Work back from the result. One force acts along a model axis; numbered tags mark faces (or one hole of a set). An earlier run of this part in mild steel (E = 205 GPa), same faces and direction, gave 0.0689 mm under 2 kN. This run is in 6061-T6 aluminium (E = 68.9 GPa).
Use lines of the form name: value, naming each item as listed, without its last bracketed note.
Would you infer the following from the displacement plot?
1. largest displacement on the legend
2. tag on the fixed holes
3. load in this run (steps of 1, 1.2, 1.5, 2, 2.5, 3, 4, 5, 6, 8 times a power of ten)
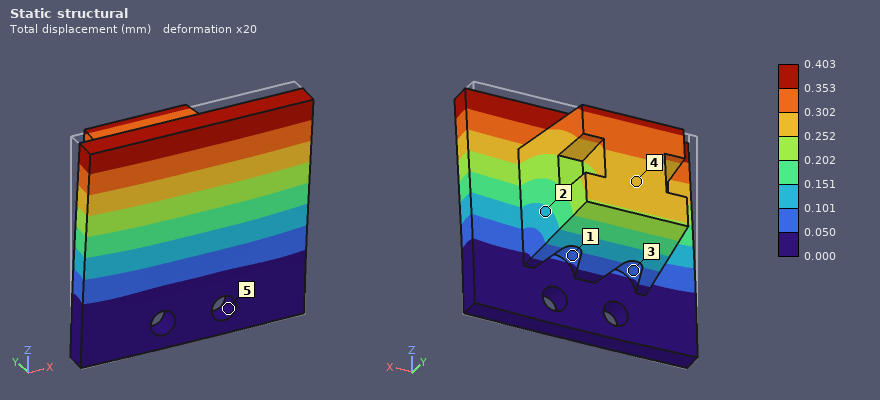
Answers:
largest displacement on the legend: 0.403 mm
tag on the fixed holes: 5
load in this run: 4 kN
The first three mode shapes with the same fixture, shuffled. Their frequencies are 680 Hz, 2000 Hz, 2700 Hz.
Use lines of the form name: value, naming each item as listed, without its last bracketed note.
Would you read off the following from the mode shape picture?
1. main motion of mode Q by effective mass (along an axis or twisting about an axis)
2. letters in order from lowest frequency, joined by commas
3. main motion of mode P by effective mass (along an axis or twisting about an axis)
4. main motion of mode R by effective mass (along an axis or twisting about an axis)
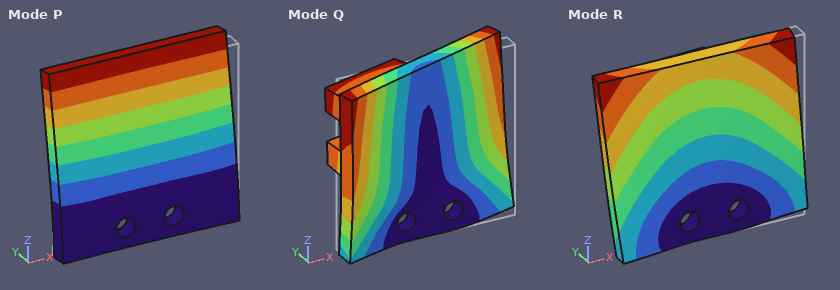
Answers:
main motion of mode Q by effective mass: along X
letters in order from lowest frequency, joined by commas: P, Q, R
main motion of mode P by effective mass: along Y
main motion of mode R by effective mass: along X
